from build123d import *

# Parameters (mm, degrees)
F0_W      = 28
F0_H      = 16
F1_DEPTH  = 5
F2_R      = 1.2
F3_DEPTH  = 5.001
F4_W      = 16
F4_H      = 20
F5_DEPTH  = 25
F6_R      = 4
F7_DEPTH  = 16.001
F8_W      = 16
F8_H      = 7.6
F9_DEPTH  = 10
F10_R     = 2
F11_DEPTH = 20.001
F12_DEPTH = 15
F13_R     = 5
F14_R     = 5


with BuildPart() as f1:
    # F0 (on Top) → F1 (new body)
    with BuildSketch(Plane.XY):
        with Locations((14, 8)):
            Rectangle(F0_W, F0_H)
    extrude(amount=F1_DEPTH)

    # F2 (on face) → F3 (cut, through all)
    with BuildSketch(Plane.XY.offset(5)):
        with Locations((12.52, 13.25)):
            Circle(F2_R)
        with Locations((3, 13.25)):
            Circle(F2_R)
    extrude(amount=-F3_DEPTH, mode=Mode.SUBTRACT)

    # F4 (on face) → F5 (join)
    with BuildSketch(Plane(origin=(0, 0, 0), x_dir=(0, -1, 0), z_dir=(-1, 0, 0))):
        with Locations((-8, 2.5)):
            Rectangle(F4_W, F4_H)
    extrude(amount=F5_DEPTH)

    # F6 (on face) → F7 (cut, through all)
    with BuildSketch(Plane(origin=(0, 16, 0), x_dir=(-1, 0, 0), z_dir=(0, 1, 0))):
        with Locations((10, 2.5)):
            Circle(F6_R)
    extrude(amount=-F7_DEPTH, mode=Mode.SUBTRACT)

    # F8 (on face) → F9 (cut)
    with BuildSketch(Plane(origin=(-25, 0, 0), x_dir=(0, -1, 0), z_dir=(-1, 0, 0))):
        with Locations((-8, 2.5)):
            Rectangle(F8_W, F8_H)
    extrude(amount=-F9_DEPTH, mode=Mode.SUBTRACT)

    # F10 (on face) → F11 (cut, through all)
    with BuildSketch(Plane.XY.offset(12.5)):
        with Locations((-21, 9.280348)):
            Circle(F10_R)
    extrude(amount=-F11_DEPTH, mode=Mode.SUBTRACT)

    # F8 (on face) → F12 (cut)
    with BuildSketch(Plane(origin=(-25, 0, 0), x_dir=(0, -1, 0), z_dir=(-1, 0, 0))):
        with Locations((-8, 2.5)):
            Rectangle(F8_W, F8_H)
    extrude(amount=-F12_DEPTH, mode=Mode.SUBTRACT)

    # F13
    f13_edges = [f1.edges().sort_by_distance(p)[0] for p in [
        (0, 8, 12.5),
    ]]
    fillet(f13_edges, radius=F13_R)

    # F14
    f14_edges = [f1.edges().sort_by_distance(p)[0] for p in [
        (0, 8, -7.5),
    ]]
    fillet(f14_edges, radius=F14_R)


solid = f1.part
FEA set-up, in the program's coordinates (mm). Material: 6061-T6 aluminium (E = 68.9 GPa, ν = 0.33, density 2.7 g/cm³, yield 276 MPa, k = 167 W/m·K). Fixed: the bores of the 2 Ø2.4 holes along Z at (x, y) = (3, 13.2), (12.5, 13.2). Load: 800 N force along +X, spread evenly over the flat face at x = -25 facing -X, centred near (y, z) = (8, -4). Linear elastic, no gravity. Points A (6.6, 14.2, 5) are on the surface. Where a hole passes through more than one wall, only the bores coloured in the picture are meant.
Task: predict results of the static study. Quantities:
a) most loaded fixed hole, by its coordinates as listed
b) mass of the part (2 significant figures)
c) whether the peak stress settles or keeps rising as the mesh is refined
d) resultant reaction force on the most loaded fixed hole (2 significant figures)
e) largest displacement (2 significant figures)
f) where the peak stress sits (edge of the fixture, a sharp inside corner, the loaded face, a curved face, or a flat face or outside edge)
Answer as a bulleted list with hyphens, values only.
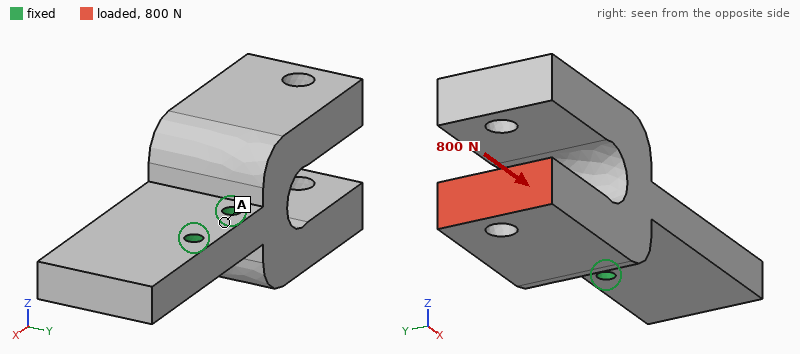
- (3, 13.2)
- 21 g
- keeps rising
- 680 N
- 0.10 mm
- edge of the fixture
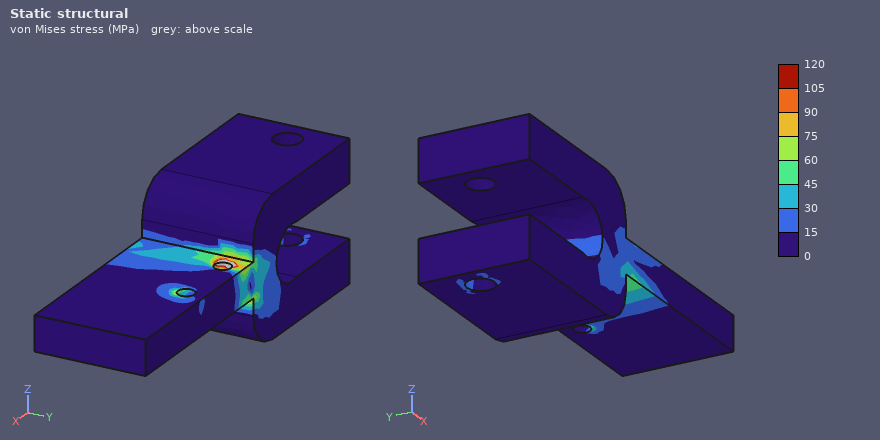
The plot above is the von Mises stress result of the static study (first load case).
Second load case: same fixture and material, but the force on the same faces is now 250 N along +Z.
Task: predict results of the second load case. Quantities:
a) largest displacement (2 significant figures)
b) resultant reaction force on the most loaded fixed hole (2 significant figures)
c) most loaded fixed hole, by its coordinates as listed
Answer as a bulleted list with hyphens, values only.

- 0.16 mm
- 500 N
- (3, 13.2)
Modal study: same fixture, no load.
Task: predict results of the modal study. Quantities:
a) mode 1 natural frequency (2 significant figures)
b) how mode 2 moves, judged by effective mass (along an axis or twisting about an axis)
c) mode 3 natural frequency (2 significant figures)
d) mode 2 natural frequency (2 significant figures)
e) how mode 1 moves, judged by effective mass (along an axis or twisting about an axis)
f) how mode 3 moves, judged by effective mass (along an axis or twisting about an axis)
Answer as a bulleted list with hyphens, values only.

- 3200 Hz
- along Y
- 7500 Hz
- 6300 Hz
- along Z
- twisting about X
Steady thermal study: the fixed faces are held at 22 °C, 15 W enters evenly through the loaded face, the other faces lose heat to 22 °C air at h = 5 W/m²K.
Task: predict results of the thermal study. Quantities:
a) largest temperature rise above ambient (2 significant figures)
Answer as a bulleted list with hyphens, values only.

- 32 K
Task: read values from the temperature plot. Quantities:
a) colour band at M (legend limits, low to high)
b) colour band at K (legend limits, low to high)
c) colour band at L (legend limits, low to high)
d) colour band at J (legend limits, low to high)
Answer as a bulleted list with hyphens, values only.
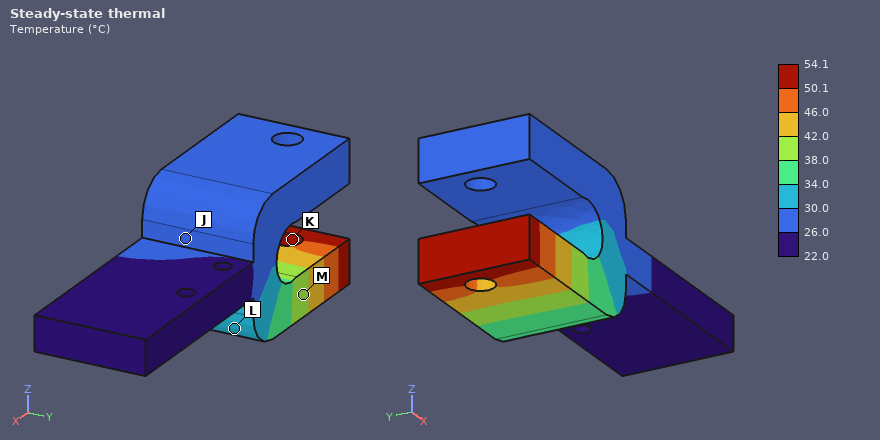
- 38.0 to 42.0 °C
- 50.1 to 54.1 °C
- 30.0 to 34.0 °C
- 26.0 to 30.0 °C
